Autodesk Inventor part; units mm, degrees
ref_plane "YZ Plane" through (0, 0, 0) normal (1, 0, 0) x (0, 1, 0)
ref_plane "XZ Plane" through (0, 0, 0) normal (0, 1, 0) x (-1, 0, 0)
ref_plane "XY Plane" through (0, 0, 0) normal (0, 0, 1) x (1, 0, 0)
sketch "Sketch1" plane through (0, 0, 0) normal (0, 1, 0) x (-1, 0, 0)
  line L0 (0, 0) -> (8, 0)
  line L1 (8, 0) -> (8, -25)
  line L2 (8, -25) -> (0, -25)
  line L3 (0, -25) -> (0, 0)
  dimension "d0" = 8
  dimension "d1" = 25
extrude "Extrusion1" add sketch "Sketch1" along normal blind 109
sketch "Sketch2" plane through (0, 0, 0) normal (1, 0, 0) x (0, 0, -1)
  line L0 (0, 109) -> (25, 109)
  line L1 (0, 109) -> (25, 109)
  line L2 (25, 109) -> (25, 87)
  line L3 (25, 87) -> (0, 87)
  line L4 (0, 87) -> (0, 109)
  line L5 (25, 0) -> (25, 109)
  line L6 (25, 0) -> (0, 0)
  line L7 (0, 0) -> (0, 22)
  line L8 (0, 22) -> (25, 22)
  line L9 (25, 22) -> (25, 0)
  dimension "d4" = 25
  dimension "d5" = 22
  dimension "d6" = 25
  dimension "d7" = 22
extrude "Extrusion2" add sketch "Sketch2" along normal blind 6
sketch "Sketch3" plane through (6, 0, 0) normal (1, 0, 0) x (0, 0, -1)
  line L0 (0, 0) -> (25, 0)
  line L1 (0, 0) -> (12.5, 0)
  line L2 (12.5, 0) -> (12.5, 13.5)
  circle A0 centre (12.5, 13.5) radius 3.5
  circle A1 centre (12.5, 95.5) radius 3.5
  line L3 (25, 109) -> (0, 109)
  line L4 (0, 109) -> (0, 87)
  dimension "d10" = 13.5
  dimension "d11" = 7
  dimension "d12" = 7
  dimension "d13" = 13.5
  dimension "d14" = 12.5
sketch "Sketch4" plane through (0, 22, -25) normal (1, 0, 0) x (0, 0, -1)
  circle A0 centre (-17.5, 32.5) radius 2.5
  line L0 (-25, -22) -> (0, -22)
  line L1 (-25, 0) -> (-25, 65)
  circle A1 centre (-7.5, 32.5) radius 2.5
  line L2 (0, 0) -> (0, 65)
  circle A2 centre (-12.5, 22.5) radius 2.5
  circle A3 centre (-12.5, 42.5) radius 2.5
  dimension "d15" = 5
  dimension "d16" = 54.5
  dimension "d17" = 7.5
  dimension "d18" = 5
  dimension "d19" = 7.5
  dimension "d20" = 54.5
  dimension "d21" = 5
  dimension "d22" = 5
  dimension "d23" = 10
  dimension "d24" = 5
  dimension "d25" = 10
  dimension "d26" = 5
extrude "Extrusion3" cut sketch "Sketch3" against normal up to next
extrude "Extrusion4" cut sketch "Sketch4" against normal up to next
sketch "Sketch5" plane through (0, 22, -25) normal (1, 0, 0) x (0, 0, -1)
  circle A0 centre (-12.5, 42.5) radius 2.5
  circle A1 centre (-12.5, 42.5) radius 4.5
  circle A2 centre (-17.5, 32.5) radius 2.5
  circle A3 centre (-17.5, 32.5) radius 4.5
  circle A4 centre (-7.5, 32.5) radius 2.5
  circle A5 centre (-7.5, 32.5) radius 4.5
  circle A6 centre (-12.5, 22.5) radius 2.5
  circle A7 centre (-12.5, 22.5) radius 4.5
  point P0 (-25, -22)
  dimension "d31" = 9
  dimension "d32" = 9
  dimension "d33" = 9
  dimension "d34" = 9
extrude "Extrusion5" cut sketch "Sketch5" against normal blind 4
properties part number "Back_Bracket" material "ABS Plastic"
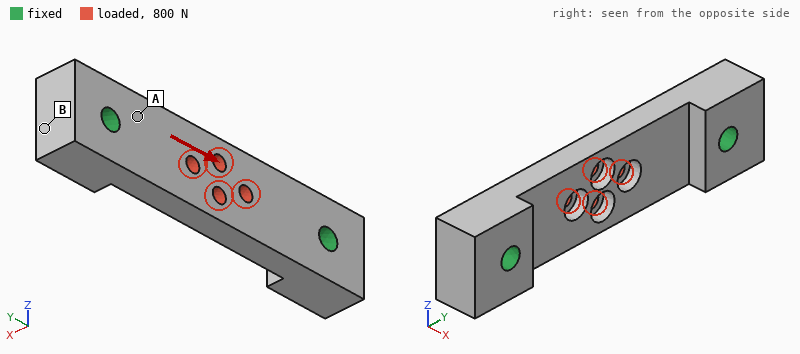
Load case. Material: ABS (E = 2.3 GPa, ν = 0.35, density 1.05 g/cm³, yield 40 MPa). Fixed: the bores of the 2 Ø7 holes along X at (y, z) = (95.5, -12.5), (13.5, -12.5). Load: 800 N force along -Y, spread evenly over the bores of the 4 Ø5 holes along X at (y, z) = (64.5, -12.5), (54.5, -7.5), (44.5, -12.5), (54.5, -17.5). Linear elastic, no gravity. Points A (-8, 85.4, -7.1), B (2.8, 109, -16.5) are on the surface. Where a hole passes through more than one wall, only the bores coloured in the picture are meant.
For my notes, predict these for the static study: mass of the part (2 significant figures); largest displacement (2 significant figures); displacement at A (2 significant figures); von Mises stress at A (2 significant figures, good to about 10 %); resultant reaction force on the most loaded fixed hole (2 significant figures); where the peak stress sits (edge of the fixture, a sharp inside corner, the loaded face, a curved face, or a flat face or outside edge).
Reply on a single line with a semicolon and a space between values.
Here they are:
27 g; 51 µm; 8.9 µm; 1.7 MPa; 400 N; the loaded face
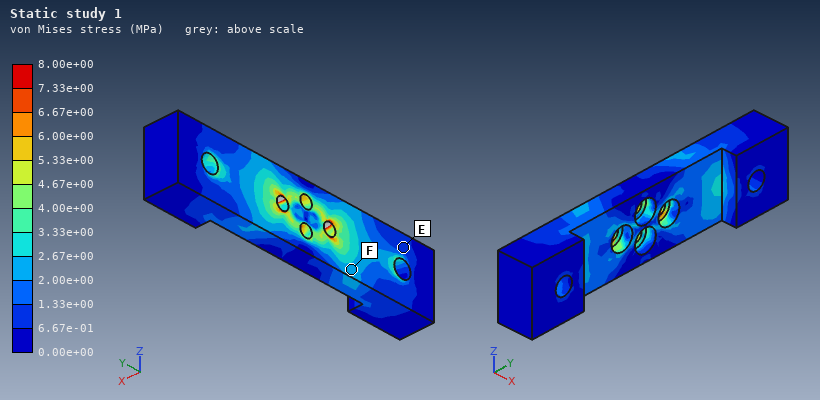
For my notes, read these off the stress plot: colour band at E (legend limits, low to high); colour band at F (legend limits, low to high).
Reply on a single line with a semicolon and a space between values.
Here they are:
6.67e-01 to 1.33e+00 MPa; 2.00e+00 to 2.67e+00 MPa
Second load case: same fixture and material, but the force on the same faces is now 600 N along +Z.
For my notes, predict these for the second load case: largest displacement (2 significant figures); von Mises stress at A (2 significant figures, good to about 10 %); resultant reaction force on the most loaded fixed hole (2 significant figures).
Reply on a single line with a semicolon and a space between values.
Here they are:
0.21 mm; 4.0 MPa; 300 N
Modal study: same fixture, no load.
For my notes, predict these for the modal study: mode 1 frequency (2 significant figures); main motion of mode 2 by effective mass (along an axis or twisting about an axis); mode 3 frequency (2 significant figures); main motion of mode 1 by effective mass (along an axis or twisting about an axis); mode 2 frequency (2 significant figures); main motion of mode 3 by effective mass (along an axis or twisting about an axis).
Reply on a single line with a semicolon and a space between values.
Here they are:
2200 Hz; along Z; 3800 Hz; along X; 3500 Hz; twisting about Y
